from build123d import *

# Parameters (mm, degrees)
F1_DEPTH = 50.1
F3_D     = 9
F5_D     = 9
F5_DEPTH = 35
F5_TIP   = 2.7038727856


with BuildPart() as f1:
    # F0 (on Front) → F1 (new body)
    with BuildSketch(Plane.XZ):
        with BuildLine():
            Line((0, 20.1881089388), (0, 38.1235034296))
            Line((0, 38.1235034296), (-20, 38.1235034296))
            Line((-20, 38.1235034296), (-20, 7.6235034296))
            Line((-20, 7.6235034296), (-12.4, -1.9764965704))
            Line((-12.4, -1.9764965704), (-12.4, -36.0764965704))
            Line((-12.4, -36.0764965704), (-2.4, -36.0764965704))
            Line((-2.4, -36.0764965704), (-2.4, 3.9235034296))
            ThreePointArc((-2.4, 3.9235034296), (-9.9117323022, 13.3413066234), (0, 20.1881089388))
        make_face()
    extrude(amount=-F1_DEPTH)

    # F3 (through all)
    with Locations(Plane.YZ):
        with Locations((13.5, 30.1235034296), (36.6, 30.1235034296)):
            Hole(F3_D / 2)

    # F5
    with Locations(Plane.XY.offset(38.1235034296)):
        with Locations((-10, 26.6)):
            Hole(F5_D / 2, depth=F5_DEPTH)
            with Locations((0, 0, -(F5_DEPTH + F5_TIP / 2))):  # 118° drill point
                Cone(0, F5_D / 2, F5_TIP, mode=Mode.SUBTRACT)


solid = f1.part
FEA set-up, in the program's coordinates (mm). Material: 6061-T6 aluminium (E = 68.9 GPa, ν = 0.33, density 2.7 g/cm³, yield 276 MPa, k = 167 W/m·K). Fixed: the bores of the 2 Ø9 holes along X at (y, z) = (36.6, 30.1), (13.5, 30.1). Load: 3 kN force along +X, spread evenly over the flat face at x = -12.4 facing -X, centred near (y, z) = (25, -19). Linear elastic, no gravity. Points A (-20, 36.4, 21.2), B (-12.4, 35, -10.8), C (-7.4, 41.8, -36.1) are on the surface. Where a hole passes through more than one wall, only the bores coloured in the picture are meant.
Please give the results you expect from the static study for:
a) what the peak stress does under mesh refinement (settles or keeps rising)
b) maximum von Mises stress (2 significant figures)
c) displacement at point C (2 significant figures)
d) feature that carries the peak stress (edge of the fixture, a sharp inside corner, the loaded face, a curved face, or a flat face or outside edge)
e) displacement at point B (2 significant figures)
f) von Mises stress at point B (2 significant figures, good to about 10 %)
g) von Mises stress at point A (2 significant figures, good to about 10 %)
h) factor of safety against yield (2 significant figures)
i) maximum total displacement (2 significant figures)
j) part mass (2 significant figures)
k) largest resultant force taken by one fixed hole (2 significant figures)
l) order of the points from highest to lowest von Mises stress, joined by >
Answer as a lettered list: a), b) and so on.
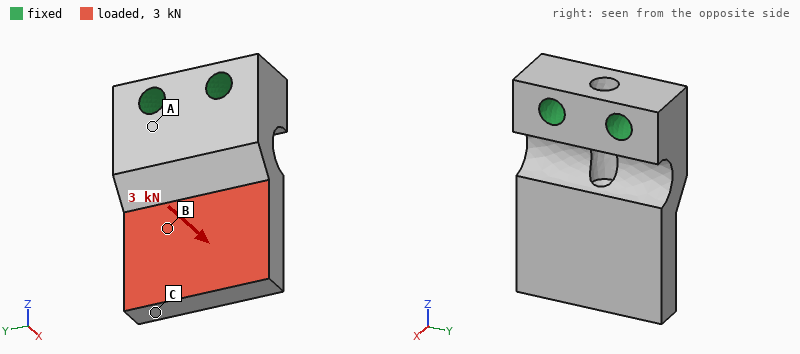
a) settles
b) 190 MPa
c) 0.46 mm
d) a curved face
e) 0.20 mm
f) 34 MPa
g) 98 MPa
h) 1.4
i) 0.47 mm
j) 120 g
k) 1.6 kN
l) A > B > C
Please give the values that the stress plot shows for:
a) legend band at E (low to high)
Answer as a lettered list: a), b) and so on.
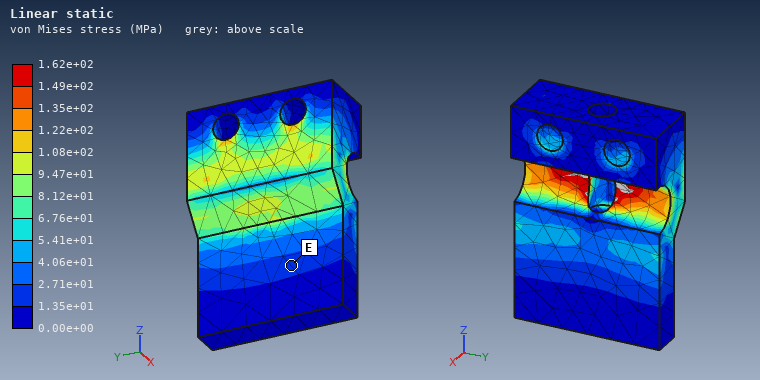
a) 1.35e+01 to 2.71e+01 MPa
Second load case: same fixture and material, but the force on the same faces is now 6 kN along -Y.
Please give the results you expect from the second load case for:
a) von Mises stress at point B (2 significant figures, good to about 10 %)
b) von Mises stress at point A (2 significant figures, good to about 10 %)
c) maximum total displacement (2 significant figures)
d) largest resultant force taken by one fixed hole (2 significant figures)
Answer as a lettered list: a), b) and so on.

a) 54 MPa
b) 37 MPa
c) 0.14 mm
d) 8.9 kN
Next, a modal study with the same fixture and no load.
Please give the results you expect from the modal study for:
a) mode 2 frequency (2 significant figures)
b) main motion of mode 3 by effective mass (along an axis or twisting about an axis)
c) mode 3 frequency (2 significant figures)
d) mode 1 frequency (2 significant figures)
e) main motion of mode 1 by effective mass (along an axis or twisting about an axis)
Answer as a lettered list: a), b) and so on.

a) 5700 Hz
b) along Y
c) 6100 Hz
d) 2200 Hz
e) along X
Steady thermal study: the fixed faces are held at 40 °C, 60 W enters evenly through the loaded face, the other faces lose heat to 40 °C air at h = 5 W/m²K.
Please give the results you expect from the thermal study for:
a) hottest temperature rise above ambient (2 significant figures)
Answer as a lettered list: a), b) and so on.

a) 35 K
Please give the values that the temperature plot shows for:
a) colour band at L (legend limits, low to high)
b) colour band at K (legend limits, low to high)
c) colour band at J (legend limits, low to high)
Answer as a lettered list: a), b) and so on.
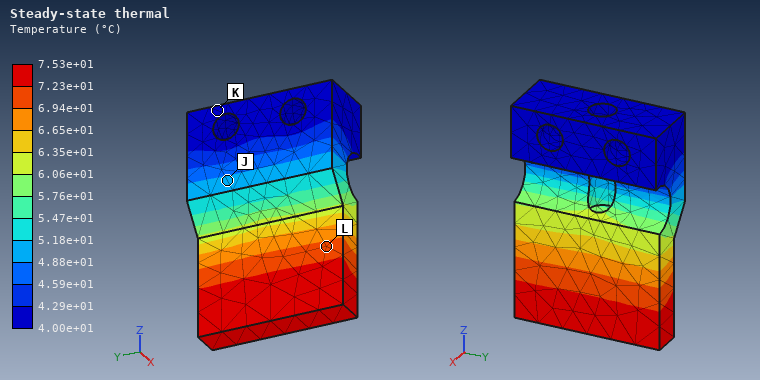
a) 6.94e+01 to 7.23e+01 °C
b) 4.00e+01 to 4.29e+01 °C
c) 4.88e+01 to 5.18e+01 °C
